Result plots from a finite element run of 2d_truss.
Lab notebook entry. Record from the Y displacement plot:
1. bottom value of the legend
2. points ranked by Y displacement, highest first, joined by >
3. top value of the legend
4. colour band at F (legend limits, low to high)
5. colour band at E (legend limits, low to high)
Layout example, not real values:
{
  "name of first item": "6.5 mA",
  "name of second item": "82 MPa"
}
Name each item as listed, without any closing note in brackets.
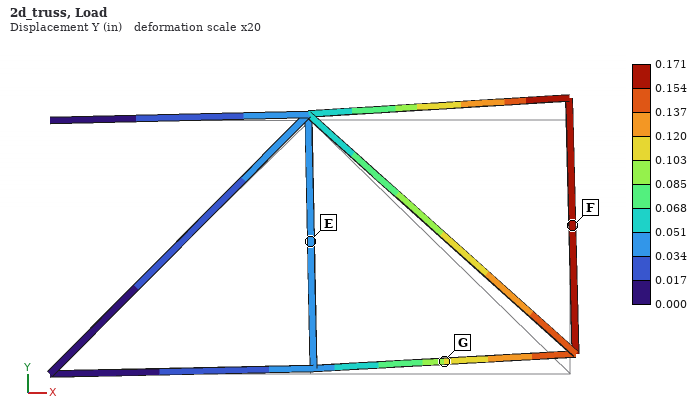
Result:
{
  "bottom value of the legend": "0.000 in",
  "points ranked by Y displacement, highest first, joined by >": "F > G > E",
  "top value of the legend": "0.171 in",
  "colour band at F": "0.154 to 0.171 in",
  "colour band at E": "0.034 to 0.051 in"
}
